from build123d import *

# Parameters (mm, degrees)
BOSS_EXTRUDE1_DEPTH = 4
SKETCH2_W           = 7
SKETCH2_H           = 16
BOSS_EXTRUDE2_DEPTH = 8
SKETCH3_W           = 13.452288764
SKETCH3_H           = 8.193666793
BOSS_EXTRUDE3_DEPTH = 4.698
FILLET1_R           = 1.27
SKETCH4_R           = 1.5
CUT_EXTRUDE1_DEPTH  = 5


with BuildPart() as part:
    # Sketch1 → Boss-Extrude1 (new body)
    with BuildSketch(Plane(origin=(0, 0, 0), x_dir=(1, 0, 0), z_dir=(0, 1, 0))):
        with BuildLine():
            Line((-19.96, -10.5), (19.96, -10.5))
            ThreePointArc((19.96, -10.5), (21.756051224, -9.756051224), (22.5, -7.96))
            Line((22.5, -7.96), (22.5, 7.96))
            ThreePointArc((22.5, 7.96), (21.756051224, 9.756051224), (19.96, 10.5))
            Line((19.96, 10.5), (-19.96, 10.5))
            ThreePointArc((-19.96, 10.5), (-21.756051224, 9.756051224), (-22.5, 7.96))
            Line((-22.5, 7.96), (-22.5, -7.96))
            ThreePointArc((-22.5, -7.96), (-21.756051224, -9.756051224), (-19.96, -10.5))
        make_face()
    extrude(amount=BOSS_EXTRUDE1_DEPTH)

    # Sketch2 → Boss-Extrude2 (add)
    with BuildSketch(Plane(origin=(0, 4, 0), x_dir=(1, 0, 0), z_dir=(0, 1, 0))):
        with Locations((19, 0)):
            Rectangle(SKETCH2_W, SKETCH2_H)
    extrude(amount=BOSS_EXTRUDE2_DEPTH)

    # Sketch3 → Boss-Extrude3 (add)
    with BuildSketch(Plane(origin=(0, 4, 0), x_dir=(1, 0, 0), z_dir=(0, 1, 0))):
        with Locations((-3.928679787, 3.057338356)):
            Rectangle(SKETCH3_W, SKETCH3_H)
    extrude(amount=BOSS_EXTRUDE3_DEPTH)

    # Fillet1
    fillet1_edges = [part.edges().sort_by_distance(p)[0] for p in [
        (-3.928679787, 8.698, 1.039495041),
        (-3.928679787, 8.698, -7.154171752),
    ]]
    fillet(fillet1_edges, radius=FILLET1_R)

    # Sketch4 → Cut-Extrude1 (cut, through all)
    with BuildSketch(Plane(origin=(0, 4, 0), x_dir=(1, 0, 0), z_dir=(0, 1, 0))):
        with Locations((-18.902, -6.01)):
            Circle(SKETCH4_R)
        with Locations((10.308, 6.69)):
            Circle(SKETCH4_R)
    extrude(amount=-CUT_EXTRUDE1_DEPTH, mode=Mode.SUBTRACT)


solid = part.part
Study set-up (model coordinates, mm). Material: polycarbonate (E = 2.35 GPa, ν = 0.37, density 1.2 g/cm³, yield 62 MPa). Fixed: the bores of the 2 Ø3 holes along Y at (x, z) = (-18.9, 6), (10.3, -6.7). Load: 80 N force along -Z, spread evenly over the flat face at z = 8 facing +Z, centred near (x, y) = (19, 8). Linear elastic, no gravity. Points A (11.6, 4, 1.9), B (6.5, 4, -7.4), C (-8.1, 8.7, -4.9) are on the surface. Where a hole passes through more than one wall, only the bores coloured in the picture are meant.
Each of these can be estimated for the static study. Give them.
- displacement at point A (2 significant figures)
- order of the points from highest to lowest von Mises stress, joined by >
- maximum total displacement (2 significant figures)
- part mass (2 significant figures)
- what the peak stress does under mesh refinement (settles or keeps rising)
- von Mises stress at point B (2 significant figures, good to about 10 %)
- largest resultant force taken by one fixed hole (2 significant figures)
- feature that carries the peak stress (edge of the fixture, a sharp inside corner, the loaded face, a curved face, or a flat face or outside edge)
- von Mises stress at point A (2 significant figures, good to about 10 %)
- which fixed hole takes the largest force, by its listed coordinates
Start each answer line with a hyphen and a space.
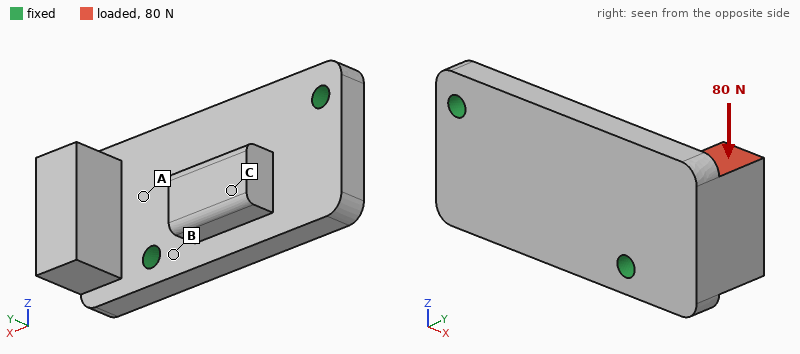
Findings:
- 0.068 mm
- A > B > C
- 0.23 mm
- 6.1 g
- keeps rising
- 2.7 MPa
- 92 N
- edge of the fixture
- 4.1 MPa
- (10.3, -6.7)
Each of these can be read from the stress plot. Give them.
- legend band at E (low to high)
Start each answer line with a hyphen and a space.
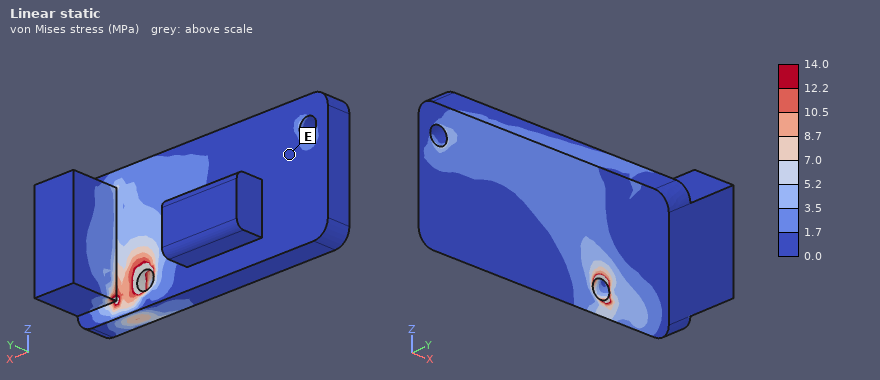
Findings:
- 0.0 to 1.7 MPa
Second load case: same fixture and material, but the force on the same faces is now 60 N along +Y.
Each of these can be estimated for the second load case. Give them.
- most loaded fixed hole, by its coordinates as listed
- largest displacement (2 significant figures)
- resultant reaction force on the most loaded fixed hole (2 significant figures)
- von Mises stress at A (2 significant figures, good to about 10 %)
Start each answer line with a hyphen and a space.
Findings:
- (10.3, -6.7)
- 0.51 mm
- 64 N
- 6.4 MPa
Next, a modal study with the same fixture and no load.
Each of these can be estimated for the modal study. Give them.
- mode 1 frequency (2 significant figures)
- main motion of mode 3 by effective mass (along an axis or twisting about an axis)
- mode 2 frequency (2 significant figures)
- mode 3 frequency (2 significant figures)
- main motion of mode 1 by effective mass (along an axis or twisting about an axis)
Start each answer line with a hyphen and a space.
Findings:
- 1900 Hz
- along Y
- 3000 Hz
- 3600 Hz
- along Y
